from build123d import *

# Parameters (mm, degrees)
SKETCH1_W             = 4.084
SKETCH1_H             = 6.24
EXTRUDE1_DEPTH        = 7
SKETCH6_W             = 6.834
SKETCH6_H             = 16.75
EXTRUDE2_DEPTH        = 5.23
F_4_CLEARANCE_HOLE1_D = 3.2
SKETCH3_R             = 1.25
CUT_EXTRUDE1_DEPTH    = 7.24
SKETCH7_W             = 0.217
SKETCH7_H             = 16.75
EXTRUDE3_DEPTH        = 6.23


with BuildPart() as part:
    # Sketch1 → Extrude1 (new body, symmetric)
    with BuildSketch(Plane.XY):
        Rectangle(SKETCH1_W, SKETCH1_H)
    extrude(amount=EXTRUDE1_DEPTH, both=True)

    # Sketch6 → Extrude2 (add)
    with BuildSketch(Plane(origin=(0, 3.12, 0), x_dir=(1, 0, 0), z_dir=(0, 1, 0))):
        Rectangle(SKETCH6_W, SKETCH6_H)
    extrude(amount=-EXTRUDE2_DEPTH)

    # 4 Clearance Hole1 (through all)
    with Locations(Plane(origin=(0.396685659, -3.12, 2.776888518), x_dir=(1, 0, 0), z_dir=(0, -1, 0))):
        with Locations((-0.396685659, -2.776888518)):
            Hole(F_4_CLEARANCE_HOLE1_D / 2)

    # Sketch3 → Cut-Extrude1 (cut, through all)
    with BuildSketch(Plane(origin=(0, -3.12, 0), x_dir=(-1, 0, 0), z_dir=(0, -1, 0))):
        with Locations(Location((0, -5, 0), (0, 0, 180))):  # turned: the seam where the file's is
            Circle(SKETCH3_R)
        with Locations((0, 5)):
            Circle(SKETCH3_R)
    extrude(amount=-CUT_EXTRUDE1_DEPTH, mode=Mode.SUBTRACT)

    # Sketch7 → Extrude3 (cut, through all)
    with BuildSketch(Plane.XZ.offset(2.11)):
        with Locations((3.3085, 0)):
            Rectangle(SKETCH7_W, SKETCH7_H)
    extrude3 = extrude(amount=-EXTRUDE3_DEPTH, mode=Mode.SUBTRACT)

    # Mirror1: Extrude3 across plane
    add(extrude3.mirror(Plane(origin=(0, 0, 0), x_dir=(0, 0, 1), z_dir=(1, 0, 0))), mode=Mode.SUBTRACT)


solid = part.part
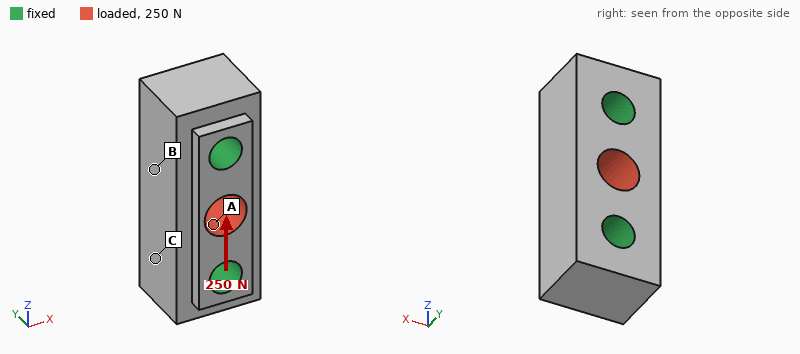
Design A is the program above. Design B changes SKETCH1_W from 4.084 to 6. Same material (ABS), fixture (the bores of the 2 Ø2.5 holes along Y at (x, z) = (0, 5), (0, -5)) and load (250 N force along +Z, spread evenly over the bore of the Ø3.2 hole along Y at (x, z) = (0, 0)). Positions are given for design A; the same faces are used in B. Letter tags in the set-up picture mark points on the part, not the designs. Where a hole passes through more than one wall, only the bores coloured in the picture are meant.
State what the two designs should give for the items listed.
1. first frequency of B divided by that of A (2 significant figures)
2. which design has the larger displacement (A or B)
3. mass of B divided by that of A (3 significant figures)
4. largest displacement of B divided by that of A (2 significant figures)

1.00
A
1.05
0.88
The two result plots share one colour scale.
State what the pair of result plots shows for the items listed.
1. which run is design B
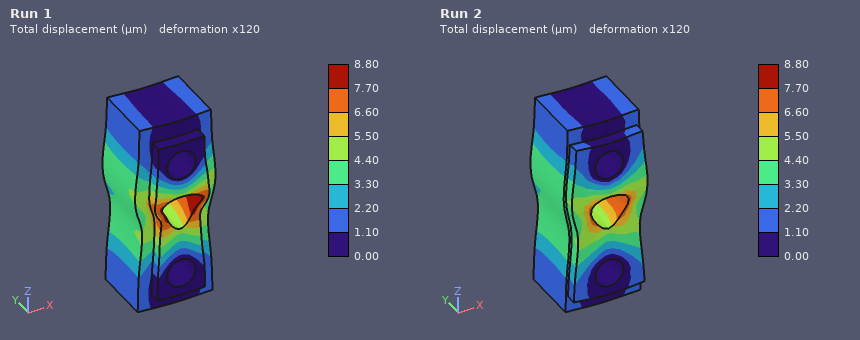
Run 2
